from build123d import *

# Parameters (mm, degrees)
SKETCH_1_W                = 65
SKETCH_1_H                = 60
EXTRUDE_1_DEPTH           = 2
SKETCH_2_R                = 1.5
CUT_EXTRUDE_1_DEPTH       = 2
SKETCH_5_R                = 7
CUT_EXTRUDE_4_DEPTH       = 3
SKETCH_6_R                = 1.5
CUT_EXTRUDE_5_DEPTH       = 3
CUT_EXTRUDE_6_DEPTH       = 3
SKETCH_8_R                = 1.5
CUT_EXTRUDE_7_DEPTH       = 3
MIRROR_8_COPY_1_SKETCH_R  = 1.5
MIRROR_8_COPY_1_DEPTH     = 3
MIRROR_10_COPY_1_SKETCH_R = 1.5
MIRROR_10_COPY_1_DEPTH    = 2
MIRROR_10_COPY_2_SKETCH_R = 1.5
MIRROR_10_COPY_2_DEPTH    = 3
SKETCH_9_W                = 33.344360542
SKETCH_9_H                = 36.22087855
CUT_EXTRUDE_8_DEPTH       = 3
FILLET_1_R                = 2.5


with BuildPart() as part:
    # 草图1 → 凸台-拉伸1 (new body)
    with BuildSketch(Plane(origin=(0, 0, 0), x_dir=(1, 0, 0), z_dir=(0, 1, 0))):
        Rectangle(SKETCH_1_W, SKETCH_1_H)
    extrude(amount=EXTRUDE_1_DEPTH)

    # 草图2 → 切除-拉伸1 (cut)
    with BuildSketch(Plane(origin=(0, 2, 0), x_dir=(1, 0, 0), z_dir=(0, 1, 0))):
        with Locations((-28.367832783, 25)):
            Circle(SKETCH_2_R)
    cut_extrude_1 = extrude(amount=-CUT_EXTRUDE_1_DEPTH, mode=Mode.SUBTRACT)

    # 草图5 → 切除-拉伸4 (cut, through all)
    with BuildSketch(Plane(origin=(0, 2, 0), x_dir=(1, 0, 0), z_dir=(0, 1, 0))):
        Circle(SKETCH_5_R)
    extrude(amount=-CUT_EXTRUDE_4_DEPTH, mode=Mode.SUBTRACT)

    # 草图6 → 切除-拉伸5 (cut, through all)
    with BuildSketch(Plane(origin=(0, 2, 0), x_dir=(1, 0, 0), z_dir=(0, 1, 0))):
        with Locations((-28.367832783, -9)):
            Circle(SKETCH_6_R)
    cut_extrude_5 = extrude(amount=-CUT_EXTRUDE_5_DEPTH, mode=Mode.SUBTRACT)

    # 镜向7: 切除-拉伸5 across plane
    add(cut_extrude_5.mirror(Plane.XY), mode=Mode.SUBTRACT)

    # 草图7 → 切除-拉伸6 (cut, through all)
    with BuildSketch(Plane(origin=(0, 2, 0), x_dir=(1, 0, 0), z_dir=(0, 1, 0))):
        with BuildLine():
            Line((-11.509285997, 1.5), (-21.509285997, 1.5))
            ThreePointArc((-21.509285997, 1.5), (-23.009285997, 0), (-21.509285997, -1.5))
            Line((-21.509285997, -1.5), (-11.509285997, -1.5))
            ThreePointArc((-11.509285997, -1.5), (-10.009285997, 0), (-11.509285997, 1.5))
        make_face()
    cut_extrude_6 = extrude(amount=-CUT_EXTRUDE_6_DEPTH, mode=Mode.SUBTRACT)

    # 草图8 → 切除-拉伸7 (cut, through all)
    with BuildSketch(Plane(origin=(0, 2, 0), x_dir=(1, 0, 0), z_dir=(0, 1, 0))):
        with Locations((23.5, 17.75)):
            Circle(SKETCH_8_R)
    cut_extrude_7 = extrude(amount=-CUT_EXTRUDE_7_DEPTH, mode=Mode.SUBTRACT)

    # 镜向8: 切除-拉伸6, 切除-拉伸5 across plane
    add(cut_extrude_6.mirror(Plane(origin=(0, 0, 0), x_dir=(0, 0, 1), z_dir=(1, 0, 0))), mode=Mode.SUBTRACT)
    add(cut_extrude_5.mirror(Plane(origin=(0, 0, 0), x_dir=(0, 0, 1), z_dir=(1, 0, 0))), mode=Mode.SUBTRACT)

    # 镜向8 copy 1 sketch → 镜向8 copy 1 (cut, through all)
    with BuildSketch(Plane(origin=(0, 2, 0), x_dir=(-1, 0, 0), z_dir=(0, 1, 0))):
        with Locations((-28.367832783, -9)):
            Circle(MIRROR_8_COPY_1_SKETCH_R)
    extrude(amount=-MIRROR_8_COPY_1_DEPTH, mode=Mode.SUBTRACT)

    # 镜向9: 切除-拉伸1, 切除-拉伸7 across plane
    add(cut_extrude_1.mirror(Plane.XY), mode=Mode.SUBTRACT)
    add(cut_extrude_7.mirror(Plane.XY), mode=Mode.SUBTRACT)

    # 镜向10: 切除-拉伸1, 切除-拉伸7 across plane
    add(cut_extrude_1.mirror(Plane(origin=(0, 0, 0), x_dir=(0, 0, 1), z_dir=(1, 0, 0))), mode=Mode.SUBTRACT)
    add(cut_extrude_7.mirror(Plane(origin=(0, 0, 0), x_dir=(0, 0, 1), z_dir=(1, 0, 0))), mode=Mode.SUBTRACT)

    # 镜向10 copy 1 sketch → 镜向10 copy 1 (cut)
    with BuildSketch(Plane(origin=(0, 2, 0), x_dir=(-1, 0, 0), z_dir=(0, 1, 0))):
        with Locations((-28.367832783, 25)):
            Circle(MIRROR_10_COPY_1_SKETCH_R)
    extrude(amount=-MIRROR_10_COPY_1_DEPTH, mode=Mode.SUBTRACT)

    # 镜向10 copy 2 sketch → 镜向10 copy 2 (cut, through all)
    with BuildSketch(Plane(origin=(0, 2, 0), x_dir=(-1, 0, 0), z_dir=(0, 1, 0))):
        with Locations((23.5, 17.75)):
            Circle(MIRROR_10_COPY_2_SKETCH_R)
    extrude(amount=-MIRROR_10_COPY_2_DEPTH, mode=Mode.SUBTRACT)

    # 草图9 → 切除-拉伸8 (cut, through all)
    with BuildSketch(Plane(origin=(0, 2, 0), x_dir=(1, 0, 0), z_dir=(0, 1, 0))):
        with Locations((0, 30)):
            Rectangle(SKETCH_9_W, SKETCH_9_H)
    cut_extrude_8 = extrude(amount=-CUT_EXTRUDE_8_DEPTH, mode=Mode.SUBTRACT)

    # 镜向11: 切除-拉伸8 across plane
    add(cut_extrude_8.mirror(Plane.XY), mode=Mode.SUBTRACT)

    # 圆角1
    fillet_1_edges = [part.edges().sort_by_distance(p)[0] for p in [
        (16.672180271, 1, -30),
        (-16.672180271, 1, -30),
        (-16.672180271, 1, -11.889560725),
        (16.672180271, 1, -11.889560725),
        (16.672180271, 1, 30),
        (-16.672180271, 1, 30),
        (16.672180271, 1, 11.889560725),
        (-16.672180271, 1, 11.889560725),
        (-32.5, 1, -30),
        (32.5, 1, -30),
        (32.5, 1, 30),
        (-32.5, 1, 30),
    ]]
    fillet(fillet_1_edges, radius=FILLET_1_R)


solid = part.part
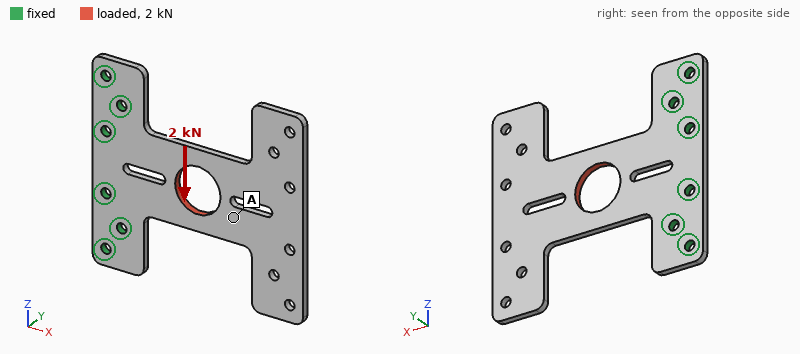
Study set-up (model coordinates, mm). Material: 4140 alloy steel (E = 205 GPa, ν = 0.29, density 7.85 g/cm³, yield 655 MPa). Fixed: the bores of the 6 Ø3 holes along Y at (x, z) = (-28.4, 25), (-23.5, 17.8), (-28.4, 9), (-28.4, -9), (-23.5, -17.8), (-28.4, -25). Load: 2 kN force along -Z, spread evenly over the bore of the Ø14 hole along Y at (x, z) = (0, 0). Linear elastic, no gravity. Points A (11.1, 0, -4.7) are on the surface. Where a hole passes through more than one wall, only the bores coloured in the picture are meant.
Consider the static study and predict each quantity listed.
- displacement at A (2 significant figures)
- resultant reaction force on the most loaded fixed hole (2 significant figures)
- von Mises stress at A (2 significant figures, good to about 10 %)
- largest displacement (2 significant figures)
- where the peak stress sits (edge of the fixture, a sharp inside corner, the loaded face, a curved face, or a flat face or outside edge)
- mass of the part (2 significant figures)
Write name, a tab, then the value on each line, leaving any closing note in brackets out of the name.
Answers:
displacement at A	0.075 mm
resultant reaction force on the most loaded fixed hole	1.2 kN
von Mises stress at A	50 MPa
largest displacement	0.10 mm
where the peak stress sits	a curved face
mass of the part	37 g
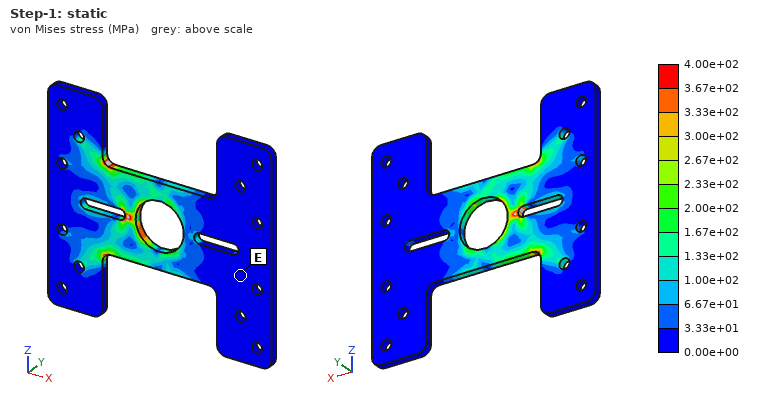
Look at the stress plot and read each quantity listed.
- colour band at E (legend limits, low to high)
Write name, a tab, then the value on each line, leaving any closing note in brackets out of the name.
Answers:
colour band at E	0.00e+00 to 3.33e+01 MPa
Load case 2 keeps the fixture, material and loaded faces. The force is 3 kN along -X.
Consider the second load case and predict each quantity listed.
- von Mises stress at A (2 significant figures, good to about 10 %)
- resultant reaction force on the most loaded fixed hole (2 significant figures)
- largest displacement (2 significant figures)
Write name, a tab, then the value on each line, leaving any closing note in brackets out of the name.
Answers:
von Mises stress at A	21 MPa
resultant reaction force on the most loaded fixed hole	1.2 kN
largest displacement	16 µm
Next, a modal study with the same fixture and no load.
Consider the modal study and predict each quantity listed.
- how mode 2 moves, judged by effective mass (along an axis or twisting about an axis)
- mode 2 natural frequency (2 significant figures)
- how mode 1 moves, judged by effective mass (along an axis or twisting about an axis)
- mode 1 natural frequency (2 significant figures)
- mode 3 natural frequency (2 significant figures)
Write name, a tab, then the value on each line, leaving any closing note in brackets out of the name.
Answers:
how mode 2 moves, judged by effective mass	twisting about X
mode 2 natural frequency	740 Hz
how mode 1 moves, judged by effective mass	along Y
mode 1 natural frequency	320 Hz
mode 3 natural frequency	2700 Hz
